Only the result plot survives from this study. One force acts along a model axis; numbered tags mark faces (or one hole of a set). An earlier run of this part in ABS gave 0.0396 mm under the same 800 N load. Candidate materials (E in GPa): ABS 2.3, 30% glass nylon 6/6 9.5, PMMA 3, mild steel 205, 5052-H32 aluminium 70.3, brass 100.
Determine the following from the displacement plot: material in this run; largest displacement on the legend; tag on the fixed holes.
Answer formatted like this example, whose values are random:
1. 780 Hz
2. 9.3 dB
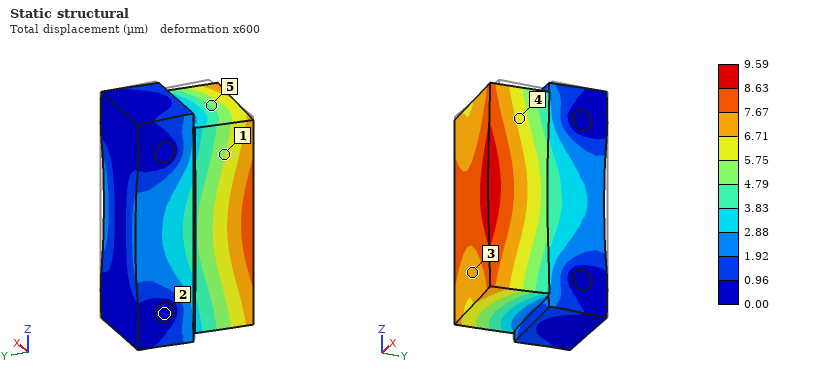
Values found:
1. 30% glass nylon 6/6
2. 9.59 µm
3. 2
